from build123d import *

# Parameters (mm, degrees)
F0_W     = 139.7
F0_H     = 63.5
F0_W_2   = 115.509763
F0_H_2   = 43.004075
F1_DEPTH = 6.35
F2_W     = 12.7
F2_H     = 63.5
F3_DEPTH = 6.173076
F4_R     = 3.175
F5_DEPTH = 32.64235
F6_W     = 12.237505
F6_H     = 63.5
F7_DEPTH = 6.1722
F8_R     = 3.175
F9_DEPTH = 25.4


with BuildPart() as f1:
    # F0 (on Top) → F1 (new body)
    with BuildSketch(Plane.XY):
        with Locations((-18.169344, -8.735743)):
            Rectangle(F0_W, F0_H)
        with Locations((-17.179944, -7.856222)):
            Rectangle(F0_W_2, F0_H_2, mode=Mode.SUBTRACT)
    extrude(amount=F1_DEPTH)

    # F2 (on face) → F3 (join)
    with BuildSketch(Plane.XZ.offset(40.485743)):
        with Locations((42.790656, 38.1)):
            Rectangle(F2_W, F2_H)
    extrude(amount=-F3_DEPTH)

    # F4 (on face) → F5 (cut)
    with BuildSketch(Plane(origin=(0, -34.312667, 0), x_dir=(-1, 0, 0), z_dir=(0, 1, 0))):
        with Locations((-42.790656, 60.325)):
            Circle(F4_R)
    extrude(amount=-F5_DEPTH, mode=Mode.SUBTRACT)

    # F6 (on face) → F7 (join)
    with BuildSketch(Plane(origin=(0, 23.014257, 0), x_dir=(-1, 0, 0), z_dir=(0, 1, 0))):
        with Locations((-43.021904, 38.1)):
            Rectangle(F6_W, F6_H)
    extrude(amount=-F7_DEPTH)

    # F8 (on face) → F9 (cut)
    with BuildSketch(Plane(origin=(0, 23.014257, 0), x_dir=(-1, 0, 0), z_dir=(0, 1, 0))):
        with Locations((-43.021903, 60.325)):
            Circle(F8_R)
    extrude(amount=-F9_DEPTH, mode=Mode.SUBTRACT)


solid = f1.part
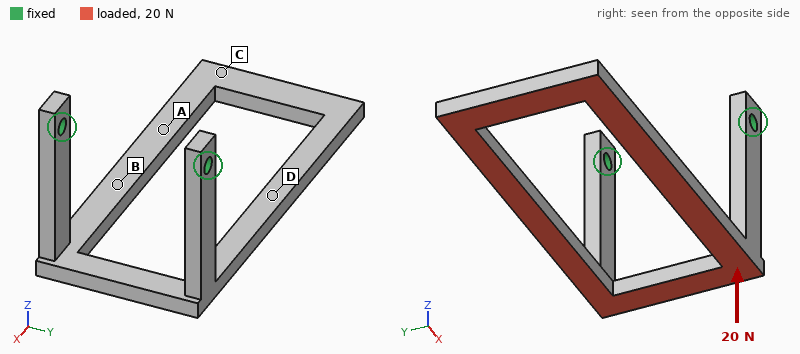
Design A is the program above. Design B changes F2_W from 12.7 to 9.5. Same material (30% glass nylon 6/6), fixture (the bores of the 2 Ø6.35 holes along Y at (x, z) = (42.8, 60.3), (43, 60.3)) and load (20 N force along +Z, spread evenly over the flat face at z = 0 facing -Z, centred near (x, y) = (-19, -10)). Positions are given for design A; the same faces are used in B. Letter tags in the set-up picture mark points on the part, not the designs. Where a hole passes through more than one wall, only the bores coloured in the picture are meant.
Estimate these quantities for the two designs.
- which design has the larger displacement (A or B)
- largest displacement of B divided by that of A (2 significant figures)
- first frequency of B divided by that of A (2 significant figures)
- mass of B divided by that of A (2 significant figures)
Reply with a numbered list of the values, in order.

1. B
2. 1.2
3. 0.92
4. 0.96
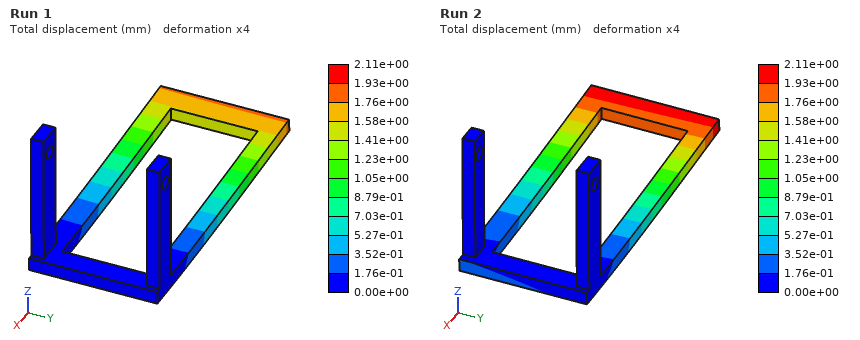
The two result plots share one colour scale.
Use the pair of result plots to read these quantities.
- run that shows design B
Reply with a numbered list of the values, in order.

1. Run 2
